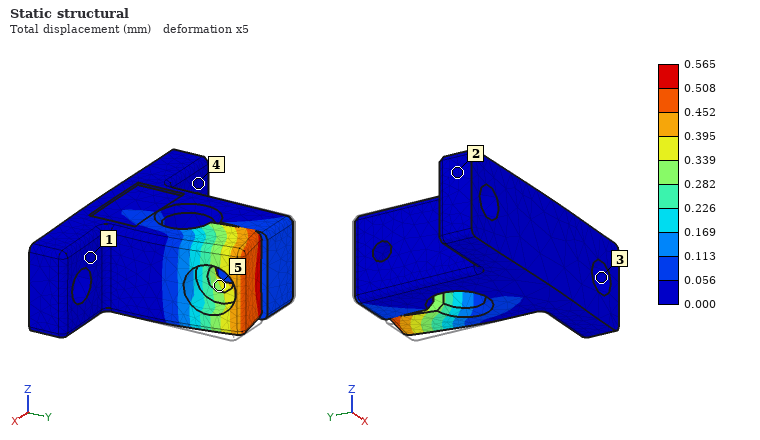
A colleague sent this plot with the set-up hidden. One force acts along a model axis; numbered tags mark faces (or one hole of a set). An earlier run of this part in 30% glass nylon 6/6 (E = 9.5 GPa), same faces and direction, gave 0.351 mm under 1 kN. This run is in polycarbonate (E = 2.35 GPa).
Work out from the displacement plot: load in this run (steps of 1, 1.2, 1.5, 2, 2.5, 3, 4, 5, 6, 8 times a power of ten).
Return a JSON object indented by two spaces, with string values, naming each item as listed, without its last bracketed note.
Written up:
{
  "load in this run": "400 N"
}
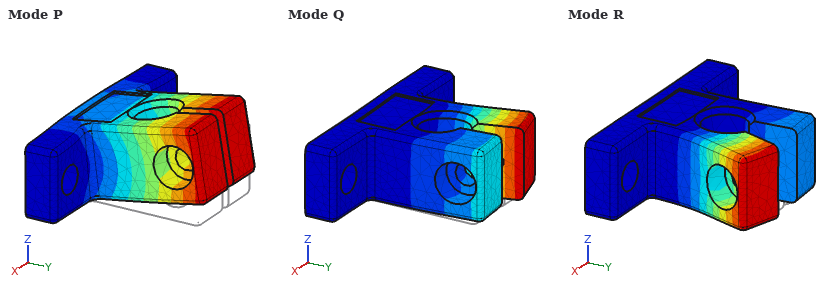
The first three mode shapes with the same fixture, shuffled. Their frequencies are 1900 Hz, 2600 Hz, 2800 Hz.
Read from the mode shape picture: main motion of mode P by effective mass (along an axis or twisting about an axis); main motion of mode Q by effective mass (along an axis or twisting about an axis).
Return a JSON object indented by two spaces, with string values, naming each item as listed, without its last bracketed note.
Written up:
{
  "main motion of mode P by effective mass": "along Z",
  "main motion of mode Q by effective mass": "along X"
}
